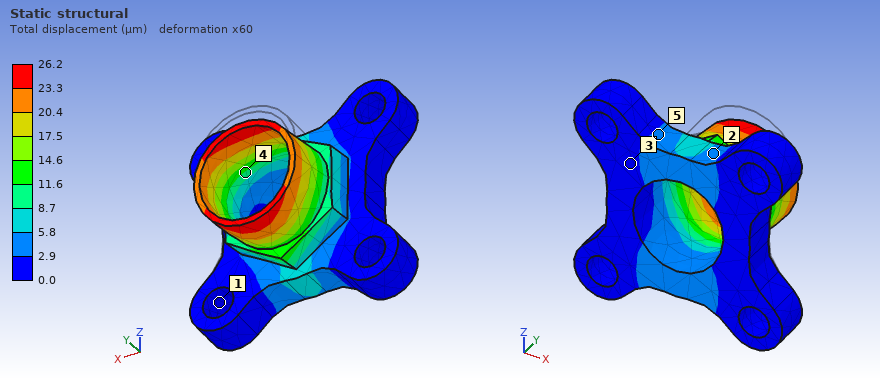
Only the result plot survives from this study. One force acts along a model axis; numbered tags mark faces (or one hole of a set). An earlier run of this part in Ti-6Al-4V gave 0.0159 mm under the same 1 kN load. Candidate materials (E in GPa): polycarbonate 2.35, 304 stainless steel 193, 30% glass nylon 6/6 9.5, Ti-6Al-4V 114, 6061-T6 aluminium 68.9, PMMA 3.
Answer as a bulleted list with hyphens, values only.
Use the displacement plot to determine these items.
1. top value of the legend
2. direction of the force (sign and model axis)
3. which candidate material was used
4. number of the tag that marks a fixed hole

- 26.2 µm
- -Z
- 6061-T6 aluminium
- 1
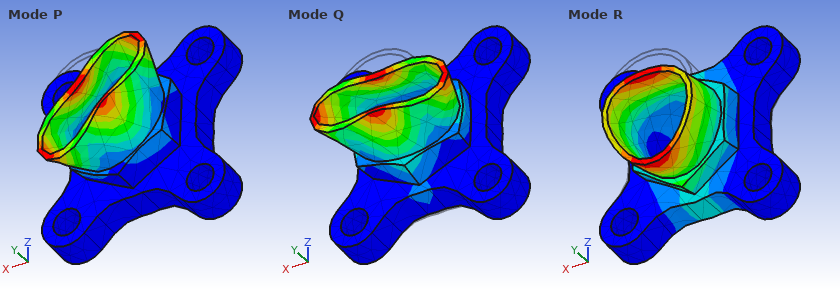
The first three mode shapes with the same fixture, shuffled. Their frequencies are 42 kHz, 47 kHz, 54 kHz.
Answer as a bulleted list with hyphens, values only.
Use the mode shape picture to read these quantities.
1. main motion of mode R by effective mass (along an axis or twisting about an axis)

- along Z
